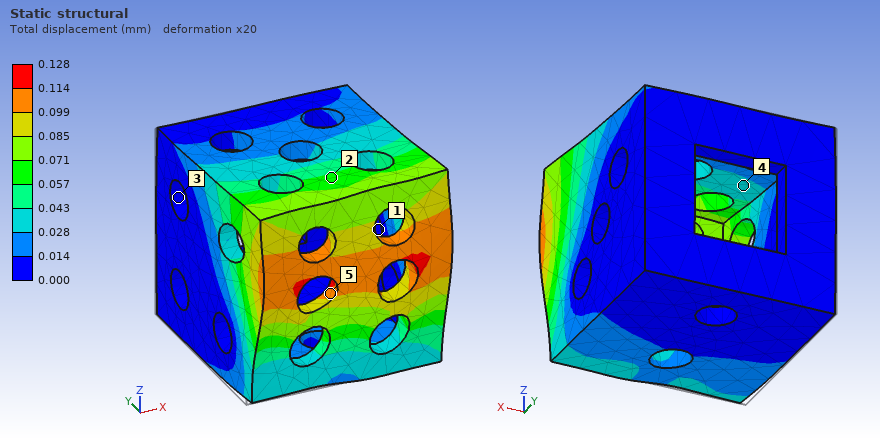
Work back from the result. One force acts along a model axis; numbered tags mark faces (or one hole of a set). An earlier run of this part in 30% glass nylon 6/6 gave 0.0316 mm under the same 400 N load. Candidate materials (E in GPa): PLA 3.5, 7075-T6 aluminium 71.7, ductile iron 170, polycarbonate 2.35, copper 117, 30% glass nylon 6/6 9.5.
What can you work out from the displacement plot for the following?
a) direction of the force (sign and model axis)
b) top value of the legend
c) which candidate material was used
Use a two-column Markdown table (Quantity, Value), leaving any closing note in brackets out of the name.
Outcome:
| Quantity | Value |
|---|---|
| direction of the force | +X |
| top value of the legend | 0.128 mm |
| which candidate material was used | polycarbonate |
